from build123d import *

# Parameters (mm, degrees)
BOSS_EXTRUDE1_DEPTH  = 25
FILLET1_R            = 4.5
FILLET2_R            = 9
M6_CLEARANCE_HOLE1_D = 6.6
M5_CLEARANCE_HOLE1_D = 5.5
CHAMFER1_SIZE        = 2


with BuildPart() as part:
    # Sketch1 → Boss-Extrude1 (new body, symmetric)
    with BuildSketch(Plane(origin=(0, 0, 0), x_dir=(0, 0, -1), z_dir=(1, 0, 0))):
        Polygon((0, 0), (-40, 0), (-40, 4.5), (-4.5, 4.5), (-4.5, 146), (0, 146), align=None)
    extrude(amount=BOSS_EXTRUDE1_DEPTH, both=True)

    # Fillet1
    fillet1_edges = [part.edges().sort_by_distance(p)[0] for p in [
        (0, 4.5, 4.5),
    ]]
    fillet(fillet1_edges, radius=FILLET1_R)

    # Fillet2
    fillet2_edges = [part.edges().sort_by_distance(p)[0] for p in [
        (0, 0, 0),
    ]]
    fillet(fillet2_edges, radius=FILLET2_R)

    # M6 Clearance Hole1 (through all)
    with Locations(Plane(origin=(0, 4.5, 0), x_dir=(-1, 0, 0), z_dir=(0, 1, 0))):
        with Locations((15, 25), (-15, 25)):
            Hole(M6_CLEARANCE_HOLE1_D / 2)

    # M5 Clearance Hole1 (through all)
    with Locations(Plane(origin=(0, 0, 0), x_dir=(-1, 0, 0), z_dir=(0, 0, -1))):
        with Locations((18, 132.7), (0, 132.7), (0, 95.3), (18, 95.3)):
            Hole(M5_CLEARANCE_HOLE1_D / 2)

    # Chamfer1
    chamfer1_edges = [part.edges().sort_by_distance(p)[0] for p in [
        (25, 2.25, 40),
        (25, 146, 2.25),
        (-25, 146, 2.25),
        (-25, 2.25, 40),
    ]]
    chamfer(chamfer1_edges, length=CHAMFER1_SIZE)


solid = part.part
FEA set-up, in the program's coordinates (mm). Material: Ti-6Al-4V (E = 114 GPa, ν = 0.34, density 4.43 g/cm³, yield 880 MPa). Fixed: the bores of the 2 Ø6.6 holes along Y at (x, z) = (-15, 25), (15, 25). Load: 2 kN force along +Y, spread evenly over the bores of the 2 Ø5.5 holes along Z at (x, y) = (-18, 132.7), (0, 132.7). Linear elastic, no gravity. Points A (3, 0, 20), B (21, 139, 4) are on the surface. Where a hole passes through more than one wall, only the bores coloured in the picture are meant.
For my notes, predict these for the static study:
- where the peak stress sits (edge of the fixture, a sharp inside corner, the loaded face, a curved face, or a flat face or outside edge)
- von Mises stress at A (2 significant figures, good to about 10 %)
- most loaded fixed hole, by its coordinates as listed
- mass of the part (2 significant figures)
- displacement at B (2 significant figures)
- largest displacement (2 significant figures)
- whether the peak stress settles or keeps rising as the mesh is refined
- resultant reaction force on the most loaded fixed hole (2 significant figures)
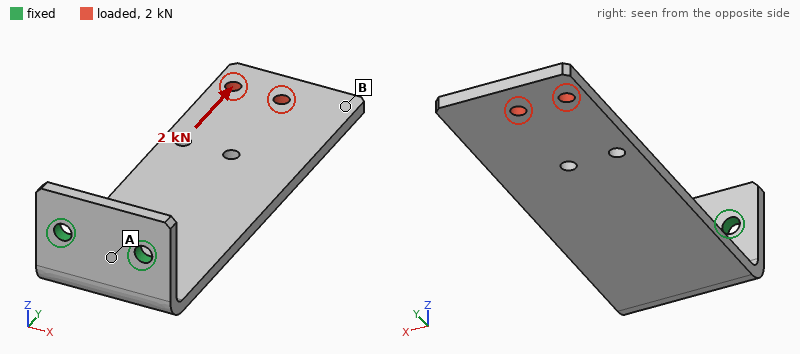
edge of the fixture
110 MPa
(-15, 25)
170 g
1.4 mm
1.6 mm
keeps rising
1.5 kN
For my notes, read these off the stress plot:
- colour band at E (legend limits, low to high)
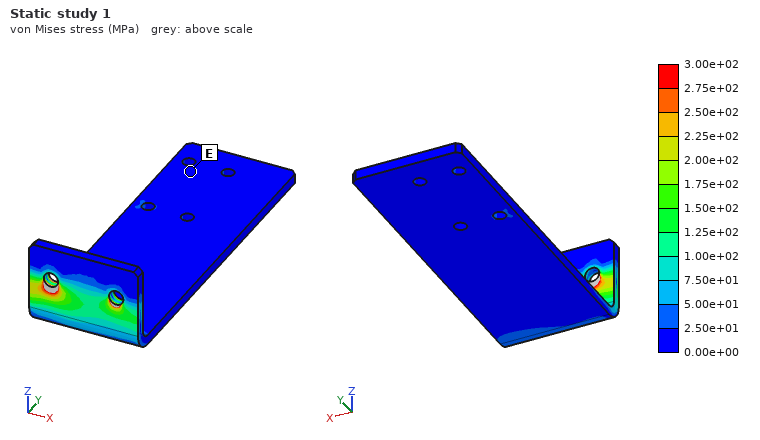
0.00e+00 to 2.50e+01 MPa
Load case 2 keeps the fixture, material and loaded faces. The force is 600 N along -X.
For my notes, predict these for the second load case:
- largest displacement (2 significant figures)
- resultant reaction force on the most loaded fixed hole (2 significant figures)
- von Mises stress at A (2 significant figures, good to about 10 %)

1.5 mm
2.3 kN
86 MPa
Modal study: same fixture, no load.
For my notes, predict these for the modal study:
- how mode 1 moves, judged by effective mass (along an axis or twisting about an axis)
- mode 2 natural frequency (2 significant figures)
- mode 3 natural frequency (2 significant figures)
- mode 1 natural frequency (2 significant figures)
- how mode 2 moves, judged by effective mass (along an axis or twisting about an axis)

along Z
450 Hz
930 Hz
150 Hz
along X
